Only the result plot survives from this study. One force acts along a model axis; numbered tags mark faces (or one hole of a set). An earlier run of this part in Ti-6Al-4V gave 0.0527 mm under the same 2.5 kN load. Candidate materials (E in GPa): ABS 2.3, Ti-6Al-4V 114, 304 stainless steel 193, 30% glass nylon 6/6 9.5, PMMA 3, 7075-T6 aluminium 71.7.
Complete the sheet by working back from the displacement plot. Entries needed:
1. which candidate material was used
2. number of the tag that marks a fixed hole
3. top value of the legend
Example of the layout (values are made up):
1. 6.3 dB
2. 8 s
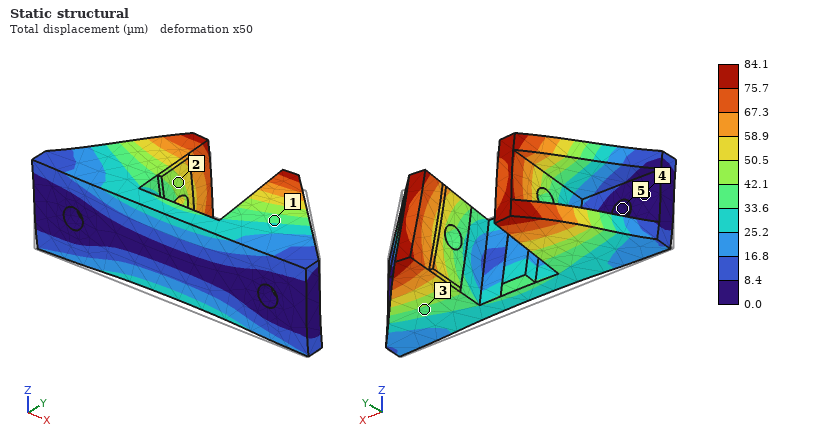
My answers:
1. 7075-T6 aluminium
2. 5
3. 84.1 µm
